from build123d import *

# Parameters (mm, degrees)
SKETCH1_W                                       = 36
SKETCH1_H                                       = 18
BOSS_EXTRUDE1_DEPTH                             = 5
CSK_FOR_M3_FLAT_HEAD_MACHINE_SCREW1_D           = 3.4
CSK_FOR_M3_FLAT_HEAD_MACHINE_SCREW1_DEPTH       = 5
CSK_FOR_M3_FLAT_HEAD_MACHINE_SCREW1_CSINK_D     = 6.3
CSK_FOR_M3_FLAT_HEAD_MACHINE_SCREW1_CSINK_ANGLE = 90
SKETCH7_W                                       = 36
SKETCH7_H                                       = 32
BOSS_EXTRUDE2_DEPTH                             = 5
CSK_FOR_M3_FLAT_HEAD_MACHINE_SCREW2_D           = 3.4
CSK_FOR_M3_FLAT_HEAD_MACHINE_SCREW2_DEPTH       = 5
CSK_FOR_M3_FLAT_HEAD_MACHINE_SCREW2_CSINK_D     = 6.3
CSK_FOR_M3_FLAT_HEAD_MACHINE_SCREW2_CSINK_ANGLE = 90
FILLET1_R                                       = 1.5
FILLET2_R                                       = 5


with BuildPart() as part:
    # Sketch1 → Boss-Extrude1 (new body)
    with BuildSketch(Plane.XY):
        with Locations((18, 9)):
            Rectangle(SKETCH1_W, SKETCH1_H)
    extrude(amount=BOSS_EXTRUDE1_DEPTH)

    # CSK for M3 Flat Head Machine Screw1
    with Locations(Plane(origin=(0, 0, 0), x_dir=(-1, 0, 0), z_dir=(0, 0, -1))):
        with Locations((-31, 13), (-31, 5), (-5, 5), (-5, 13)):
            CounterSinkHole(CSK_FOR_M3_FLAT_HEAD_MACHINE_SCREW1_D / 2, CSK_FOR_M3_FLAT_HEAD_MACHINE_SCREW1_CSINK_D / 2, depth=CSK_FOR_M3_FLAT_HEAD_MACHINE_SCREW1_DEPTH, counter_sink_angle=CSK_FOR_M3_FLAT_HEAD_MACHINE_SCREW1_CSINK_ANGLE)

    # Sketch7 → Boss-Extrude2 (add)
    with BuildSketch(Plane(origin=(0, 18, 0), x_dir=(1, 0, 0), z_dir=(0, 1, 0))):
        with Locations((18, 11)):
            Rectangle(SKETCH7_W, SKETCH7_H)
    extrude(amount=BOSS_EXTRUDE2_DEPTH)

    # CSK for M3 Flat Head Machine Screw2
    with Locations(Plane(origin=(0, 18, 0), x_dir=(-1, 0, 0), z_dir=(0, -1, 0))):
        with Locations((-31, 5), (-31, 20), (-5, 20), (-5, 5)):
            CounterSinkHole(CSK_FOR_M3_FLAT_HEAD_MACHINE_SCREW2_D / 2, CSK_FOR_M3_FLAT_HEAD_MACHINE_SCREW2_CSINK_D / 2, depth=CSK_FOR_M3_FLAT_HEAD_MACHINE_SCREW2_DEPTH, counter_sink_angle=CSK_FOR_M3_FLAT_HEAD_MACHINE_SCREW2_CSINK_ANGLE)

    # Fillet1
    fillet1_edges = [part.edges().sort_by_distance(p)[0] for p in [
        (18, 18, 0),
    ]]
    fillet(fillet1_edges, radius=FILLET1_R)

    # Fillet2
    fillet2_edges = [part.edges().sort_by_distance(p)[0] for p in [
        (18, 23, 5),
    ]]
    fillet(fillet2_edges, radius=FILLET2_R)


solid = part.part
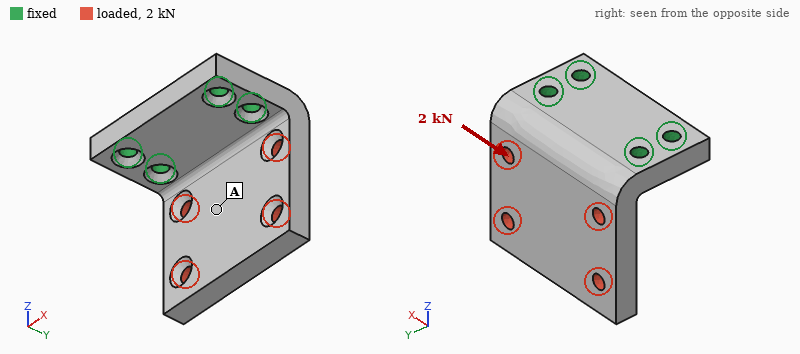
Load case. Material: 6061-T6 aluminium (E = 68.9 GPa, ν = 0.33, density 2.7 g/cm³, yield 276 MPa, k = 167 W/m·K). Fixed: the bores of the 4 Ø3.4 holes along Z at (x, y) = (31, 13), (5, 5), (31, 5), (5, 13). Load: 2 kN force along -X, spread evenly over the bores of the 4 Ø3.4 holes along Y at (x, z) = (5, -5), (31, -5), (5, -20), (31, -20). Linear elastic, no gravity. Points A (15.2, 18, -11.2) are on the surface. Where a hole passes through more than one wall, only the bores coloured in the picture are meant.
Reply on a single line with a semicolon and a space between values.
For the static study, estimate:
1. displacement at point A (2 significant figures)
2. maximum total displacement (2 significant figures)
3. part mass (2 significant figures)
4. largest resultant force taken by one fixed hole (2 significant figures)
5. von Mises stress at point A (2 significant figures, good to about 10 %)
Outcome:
27 µm; 59 µm; 23 g; 1.6 kN; 20 MPa
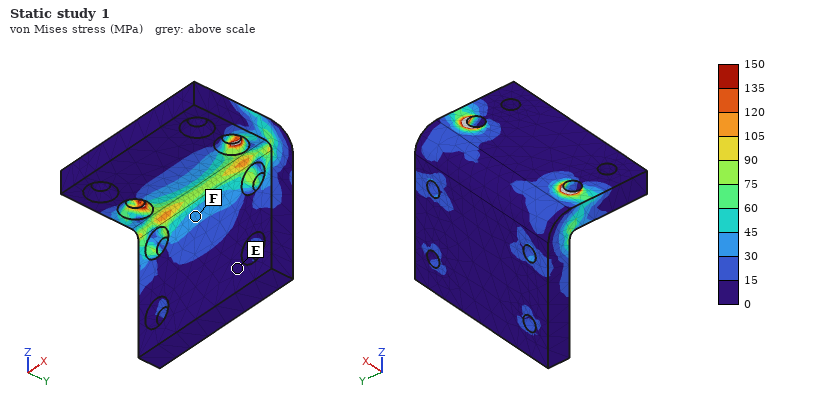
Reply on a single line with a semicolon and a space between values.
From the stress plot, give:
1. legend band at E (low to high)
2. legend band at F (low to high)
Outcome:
0 to 15 MPa; 30 to 45 MPa
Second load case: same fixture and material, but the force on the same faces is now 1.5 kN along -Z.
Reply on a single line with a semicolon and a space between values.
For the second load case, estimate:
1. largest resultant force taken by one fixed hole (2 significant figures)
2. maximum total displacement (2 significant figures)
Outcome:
1.0 kN; 99 µm
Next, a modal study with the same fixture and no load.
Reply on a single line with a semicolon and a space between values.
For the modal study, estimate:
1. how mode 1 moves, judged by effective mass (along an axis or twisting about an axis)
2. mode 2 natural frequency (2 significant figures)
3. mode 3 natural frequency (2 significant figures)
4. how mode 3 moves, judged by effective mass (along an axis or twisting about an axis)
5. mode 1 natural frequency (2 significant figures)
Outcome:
along Y; 7500 Hz; 11 kHz; along X; 3300 Hz
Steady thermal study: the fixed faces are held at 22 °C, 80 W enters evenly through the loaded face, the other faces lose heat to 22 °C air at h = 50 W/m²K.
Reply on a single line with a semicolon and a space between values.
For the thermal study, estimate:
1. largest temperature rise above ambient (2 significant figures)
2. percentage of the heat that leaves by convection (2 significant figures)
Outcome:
65 K; 8.0 %
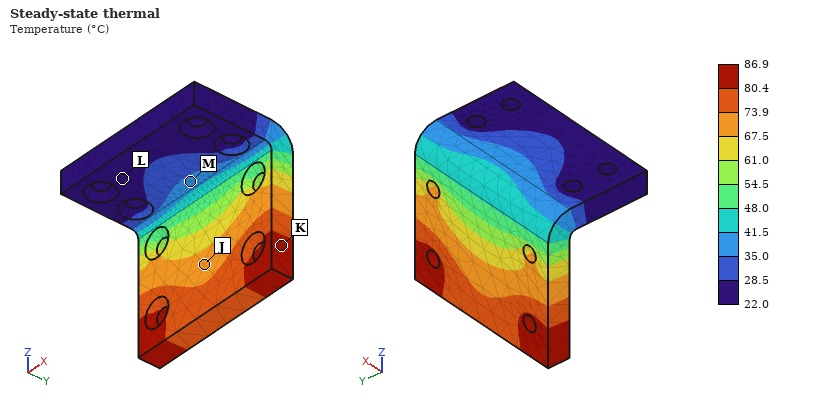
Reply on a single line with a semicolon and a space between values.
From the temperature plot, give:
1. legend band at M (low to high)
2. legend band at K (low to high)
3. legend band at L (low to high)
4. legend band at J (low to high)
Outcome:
35.0 to 41.5 °C; 80.4 to 86.9 °C; 22.0 to 28.5 °C; 67.5 to 73.9 °C
